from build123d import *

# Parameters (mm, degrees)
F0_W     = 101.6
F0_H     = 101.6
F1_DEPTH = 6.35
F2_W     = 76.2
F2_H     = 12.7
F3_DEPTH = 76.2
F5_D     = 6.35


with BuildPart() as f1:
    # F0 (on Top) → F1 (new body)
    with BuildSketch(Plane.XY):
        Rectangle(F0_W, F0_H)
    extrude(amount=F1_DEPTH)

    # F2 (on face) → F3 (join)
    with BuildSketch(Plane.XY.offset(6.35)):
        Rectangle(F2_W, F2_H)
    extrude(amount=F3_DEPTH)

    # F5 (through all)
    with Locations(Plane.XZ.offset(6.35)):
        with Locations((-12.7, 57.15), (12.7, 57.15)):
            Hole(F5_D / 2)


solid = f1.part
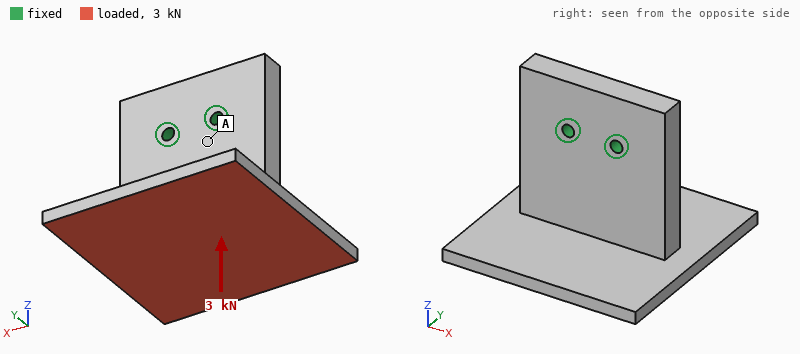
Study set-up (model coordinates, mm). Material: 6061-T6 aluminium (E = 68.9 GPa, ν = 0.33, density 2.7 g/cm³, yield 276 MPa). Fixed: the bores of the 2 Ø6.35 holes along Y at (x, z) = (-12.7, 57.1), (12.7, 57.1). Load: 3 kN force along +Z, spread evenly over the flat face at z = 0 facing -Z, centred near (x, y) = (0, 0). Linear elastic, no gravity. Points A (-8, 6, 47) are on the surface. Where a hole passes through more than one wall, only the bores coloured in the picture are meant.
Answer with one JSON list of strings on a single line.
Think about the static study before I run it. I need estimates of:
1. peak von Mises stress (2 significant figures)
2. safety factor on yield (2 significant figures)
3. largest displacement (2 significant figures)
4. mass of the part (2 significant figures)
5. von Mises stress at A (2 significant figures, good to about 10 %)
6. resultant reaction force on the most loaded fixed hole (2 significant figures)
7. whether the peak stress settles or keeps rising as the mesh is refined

["40 MPa", "6.9", "0.12 mm", "370 g", "4.1 MPa", "1.5 kN", "settles"]
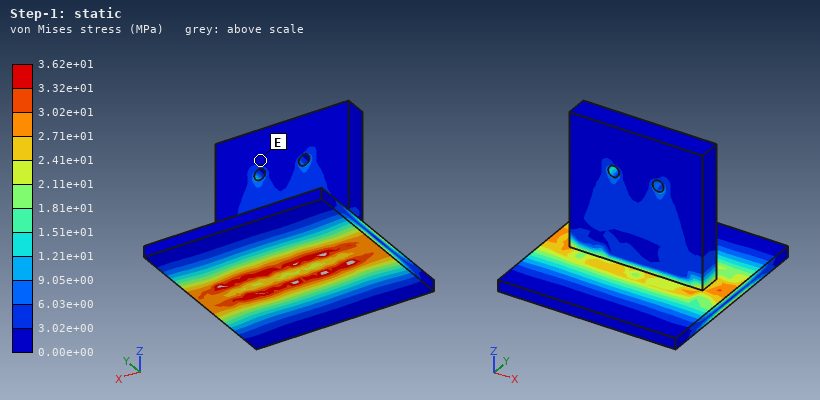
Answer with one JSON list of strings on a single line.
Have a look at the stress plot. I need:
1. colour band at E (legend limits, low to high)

["0.00e+00 to 3.02e+00 MPa"]
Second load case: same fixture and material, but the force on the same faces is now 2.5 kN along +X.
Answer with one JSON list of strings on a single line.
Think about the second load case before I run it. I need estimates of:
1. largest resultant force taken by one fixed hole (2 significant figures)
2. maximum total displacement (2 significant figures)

["4.9 kN", "39 µm"]
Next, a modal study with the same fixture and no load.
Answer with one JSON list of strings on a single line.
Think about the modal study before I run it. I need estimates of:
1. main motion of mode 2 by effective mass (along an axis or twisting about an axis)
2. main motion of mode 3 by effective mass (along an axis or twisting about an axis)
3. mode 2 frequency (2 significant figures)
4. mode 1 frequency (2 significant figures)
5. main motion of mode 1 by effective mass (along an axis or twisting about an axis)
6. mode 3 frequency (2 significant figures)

["twisting about Z", "along Z", "1500 Hz", "1000 Hz", "along Y", "2300 Hz"]
